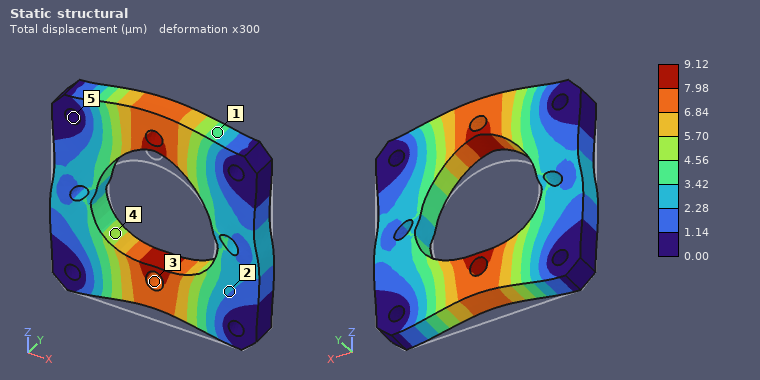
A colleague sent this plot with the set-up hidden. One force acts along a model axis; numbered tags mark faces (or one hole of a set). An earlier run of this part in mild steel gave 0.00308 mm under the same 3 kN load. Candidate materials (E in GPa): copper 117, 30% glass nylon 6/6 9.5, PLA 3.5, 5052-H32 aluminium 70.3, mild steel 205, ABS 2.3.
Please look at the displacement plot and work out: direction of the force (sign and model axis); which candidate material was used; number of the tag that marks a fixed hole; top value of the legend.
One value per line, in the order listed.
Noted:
+Z
5052-H32 aluminium
5
9.12 µm
